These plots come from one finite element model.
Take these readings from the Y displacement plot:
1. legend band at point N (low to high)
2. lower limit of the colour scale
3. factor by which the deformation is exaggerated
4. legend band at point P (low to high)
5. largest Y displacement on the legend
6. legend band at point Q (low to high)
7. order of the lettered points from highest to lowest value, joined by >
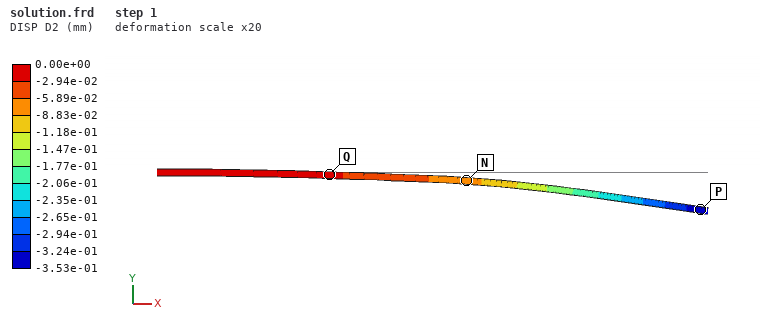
-8.83e-02 to -5.89e-02 mm
-3.53e-01 mm
20
-3.53e-01 to -3.24e-01 mm
0.00e+00 mm
-2.94e-02 to 0.00e+00 mm
Q > N > P
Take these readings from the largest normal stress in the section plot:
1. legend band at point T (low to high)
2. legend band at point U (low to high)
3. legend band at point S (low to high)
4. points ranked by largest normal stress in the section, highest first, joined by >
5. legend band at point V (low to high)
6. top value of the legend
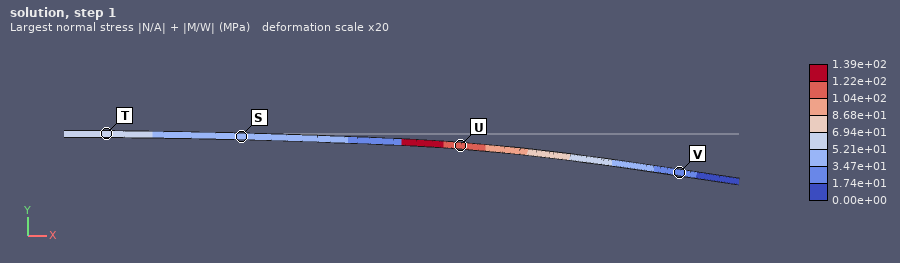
5.21e+01 to 6.94e+01 MPa
1.04e+02 to 1.22e+02 MPa
3.47e+01 to 5.21e+01 MPa
U > T > S > V
1.74e+01 to 3.47e+01 MPa
1.39e+02 MPa
